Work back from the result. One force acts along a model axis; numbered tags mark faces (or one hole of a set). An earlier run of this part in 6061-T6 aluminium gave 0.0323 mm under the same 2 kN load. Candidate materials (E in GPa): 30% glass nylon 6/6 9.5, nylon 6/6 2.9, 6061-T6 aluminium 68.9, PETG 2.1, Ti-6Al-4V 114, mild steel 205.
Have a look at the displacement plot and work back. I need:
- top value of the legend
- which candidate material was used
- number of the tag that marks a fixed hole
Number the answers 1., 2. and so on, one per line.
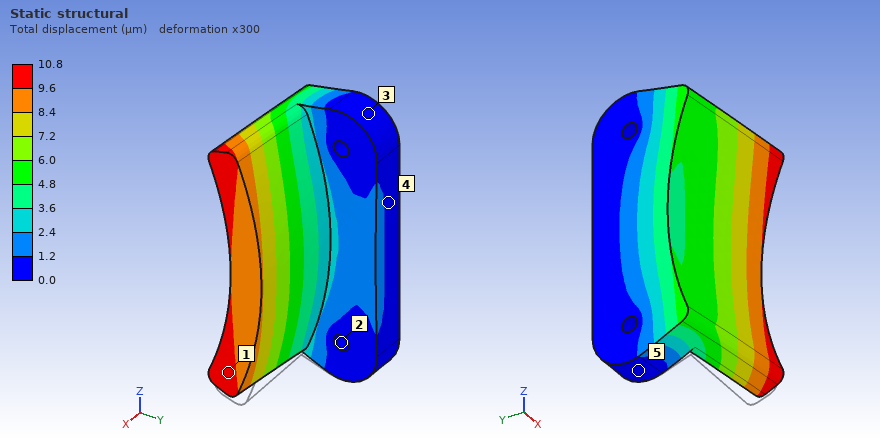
1. 10.8 µm
2. mild steel
3. 2
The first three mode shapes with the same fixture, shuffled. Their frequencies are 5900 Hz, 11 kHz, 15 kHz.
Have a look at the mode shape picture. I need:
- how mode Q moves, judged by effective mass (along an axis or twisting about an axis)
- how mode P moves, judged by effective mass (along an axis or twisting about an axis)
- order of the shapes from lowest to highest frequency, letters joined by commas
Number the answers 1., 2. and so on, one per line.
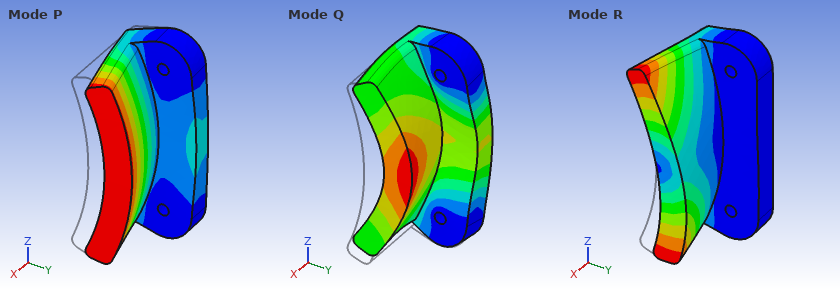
1. along X
2. along Y
3. P, R, Q
